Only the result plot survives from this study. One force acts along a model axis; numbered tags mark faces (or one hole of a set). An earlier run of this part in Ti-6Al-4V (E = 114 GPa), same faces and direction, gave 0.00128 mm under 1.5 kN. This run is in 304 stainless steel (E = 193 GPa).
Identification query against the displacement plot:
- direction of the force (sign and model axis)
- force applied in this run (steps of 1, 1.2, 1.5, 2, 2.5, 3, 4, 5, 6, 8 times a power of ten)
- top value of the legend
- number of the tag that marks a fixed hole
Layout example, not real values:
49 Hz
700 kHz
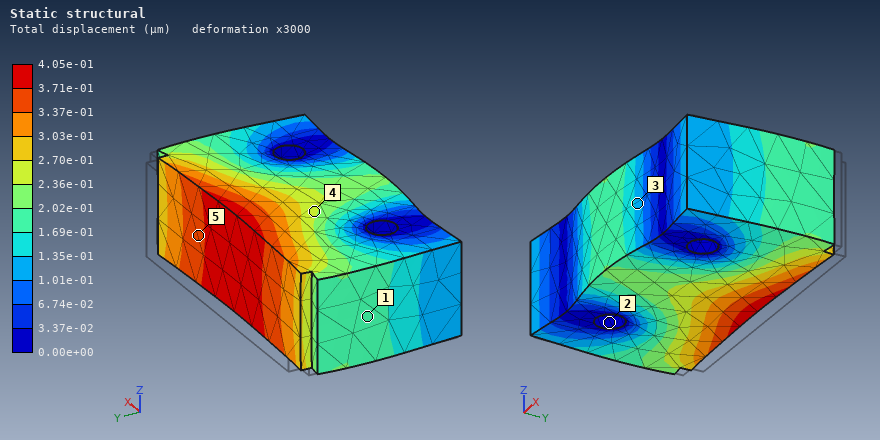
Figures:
-Y
800 N
4.05e-01 µm
2
